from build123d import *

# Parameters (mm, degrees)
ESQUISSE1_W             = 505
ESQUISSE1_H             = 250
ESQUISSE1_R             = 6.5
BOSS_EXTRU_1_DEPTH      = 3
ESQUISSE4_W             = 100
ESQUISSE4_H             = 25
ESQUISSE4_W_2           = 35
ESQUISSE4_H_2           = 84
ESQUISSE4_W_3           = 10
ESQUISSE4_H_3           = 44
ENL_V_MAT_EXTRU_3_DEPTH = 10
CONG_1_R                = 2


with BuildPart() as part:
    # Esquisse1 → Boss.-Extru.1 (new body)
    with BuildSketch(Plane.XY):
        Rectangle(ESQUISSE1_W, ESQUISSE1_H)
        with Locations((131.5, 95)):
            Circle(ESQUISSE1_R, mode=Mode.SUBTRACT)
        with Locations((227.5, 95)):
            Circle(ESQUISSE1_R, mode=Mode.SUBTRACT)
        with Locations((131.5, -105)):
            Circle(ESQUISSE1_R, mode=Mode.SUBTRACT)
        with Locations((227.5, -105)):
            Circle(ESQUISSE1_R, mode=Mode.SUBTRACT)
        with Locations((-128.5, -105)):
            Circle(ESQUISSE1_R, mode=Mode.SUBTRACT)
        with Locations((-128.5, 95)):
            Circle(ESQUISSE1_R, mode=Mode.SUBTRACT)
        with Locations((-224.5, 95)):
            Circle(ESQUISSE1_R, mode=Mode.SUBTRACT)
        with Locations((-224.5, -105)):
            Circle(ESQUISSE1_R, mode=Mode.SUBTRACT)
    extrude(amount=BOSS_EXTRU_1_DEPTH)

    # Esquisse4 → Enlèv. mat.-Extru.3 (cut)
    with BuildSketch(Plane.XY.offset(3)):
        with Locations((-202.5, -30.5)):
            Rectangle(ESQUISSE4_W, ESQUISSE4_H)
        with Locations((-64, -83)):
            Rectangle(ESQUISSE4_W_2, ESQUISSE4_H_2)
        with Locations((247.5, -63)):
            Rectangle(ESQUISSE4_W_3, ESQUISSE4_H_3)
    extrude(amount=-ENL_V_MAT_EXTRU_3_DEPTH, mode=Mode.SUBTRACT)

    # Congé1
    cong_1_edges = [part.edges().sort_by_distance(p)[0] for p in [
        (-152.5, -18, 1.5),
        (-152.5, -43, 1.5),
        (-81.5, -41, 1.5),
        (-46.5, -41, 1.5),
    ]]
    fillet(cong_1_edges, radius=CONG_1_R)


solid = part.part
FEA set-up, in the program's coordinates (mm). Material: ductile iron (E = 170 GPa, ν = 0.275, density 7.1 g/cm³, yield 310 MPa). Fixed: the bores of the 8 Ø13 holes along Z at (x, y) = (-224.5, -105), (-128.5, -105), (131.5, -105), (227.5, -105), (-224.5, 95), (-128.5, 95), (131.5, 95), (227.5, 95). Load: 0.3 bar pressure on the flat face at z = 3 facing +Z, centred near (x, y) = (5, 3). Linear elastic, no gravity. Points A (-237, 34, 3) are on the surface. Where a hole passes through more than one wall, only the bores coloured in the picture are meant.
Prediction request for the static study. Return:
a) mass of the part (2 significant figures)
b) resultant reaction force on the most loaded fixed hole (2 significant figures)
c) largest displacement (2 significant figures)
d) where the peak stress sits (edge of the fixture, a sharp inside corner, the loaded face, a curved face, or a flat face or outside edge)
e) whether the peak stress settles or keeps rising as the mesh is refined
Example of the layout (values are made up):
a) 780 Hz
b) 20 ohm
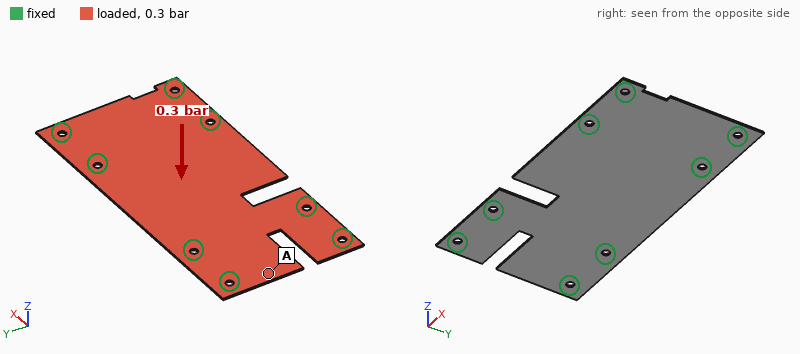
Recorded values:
a) 2.5 kg
b) 740 N
c) 2.4 mm
d) edge of the fixture
e) keeps rising
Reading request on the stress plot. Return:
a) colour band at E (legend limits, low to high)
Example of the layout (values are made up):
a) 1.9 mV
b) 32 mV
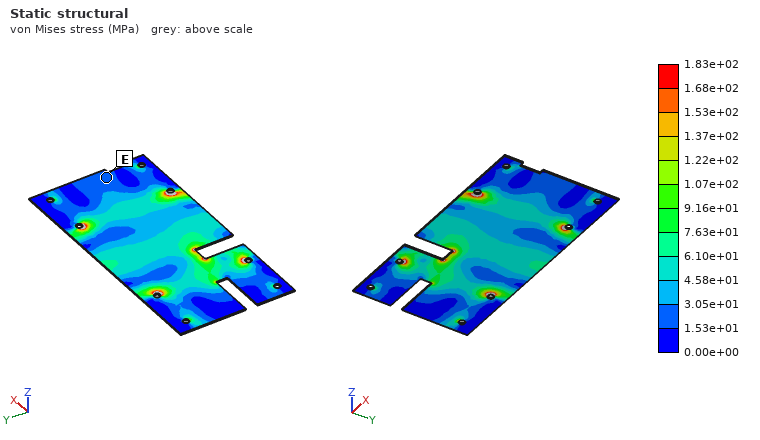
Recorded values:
a) 1.53e+01 to 3.05e+01 MPa
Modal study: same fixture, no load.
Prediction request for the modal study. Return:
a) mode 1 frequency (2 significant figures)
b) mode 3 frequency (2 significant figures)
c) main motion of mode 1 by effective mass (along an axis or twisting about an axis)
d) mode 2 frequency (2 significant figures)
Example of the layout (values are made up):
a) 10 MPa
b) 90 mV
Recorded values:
a) 160 Hz
b) 300 Hz
c) along Z
d) 240 Hz
